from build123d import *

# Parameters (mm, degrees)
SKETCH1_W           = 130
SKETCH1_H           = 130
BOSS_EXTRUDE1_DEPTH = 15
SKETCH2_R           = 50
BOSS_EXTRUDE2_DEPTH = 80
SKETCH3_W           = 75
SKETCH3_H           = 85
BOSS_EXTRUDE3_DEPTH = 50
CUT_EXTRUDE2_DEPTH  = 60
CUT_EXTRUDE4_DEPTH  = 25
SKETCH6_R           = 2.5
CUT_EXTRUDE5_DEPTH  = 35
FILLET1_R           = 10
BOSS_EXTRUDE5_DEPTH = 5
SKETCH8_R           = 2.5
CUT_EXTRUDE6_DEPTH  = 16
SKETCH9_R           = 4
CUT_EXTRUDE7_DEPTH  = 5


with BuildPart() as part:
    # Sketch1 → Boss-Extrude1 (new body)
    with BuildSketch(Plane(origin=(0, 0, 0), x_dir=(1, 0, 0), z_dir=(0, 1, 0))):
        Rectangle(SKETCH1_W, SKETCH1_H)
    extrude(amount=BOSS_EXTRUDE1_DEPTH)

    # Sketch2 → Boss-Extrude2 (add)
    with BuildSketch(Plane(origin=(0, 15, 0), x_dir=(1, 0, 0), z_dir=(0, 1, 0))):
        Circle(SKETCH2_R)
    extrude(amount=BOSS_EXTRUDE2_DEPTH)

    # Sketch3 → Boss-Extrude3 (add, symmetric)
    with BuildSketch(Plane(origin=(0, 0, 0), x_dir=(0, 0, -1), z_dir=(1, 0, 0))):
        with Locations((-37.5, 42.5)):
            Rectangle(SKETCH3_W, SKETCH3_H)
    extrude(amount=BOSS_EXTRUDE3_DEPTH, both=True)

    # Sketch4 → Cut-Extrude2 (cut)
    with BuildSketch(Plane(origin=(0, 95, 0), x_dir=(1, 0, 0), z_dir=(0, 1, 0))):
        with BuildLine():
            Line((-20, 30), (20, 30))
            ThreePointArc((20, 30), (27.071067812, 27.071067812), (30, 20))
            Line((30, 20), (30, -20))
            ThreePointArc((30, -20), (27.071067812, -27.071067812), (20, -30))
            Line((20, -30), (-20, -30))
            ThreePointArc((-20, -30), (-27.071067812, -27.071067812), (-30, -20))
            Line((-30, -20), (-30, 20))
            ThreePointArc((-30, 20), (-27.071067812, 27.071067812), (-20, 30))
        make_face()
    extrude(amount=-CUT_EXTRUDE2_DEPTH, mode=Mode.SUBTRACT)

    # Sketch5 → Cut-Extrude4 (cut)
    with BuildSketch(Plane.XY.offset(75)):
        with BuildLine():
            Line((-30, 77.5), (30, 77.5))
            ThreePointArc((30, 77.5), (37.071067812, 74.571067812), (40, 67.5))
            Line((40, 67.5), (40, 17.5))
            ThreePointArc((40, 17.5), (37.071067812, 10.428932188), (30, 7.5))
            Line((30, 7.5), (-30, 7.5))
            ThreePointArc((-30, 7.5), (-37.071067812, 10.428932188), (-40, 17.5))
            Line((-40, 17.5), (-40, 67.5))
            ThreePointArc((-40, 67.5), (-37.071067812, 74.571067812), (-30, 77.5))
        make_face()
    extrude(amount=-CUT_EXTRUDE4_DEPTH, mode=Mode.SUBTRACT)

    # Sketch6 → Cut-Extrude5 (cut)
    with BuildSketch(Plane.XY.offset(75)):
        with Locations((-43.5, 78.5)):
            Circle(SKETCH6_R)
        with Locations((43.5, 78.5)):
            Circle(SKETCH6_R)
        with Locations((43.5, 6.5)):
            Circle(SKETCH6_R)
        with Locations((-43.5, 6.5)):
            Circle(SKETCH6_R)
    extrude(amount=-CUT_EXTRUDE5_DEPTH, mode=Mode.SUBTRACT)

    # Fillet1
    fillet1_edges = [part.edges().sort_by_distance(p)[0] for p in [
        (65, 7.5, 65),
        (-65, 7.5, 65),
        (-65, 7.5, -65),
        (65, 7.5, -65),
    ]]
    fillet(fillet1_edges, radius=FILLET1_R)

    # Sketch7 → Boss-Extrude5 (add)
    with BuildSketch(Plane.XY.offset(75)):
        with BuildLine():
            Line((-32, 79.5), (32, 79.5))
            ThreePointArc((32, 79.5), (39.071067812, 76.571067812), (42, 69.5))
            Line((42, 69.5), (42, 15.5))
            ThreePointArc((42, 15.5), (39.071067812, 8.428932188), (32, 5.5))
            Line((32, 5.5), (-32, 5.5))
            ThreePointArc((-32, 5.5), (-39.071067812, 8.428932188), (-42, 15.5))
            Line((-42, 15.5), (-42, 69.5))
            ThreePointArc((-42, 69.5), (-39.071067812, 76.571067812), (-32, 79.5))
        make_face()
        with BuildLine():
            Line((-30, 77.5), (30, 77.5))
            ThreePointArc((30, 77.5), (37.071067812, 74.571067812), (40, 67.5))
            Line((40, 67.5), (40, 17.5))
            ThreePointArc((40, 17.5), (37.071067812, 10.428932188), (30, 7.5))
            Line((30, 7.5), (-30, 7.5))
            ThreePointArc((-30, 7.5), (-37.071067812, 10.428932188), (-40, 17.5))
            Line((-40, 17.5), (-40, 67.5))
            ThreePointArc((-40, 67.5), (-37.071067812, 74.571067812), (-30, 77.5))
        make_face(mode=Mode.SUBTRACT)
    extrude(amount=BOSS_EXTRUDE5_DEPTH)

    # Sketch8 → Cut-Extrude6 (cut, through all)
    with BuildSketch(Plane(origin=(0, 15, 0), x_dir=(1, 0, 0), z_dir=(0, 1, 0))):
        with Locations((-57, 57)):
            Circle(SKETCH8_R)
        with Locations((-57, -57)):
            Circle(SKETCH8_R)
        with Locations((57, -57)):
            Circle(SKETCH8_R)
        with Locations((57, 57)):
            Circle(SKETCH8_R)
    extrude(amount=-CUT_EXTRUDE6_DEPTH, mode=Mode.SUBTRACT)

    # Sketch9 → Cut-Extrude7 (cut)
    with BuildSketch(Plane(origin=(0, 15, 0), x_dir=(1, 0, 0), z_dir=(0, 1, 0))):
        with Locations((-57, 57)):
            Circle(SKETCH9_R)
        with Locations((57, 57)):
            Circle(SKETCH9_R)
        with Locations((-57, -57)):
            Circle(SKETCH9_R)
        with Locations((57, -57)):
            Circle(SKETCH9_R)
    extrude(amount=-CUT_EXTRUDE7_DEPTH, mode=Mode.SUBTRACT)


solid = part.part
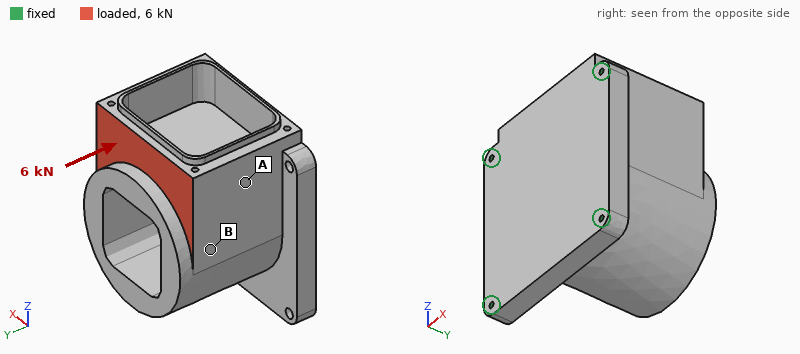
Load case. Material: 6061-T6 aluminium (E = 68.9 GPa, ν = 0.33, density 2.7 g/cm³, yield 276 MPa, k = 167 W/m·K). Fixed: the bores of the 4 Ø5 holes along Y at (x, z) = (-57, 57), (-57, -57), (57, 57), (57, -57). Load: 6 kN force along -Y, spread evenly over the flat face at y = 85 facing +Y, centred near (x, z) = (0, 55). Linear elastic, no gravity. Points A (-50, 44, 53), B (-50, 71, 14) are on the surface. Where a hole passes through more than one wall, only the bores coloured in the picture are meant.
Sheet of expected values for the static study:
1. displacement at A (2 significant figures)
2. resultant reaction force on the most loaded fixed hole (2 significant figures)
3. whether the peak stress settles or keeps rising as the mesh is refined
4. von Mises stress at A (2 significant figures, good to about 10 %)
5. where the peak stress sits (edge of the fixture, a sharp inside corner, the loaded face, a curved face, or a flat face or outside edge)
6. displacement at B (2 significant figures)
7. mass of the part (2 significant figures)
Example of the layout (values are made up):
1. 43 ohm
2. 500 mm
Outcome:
1. 11 µm
2. 3.1 kN
3. keeps rising
4. 4.5 MPa
5. edge of the fixture
6. 8.6 µm
7. 2.1 kg
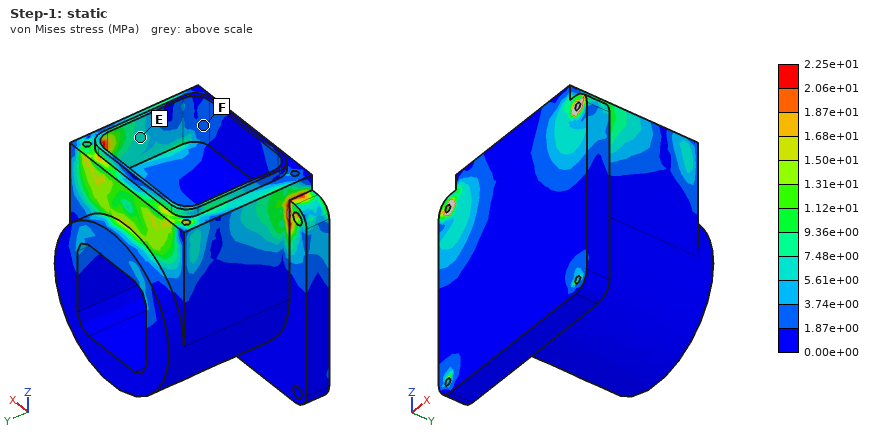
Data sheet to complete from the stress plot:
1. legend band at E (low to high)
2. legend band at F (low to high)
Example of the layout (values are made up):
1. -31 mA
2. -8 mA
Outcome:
1. 5.61e+00 to 7.48e+00 MPa
2. 1.87e+00 to 3.74e+00 MPa
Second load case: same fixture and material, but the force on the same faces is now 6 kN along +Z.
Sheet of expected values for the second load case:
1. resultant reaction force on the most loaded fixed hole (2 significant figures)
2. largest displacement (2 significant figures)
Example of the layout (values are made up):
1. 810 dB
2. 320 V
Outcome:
1. 3.1 kN
2. 48 µm
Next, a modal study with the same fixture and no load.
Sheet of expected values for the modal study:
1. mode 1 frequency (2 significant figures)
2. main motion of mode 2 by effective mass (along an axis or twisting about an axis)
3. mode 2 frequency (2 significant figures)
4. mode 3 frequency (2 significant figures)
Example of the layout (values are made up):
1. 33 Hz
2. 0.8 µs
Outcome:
1. 2100 Hz
2. along X
3. 2700 Hz
4. 3300 Hz
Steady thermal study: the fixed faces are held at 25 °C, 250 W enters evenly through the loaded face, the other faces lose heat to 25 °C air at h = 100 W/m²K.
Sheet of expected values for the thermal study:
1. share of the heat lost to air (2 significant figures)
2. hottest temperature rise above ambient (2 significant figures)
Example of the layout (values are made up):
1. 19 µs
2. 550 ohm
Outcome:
1. 56 %
2. 46 K
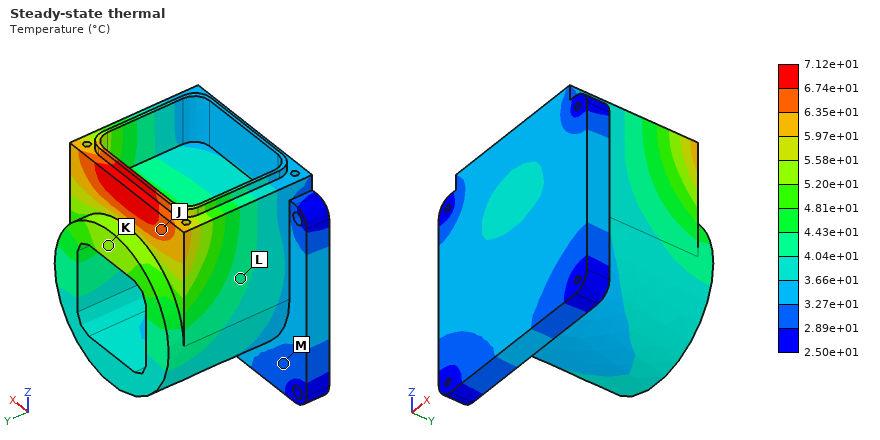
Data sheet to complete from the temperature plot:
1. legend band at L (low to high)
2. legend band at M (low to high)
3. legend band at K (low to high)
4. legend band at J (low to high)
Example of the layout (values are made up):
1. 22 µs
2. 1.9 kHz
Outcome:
1. 4.04e+01 to 4.43e+01 °C
2. 2.89e+01 to 3.27e+01 °C
3. 5.20e+01 to 5.58e+01 °C
4. 6.35e+01 to 6.74e+01 °C
